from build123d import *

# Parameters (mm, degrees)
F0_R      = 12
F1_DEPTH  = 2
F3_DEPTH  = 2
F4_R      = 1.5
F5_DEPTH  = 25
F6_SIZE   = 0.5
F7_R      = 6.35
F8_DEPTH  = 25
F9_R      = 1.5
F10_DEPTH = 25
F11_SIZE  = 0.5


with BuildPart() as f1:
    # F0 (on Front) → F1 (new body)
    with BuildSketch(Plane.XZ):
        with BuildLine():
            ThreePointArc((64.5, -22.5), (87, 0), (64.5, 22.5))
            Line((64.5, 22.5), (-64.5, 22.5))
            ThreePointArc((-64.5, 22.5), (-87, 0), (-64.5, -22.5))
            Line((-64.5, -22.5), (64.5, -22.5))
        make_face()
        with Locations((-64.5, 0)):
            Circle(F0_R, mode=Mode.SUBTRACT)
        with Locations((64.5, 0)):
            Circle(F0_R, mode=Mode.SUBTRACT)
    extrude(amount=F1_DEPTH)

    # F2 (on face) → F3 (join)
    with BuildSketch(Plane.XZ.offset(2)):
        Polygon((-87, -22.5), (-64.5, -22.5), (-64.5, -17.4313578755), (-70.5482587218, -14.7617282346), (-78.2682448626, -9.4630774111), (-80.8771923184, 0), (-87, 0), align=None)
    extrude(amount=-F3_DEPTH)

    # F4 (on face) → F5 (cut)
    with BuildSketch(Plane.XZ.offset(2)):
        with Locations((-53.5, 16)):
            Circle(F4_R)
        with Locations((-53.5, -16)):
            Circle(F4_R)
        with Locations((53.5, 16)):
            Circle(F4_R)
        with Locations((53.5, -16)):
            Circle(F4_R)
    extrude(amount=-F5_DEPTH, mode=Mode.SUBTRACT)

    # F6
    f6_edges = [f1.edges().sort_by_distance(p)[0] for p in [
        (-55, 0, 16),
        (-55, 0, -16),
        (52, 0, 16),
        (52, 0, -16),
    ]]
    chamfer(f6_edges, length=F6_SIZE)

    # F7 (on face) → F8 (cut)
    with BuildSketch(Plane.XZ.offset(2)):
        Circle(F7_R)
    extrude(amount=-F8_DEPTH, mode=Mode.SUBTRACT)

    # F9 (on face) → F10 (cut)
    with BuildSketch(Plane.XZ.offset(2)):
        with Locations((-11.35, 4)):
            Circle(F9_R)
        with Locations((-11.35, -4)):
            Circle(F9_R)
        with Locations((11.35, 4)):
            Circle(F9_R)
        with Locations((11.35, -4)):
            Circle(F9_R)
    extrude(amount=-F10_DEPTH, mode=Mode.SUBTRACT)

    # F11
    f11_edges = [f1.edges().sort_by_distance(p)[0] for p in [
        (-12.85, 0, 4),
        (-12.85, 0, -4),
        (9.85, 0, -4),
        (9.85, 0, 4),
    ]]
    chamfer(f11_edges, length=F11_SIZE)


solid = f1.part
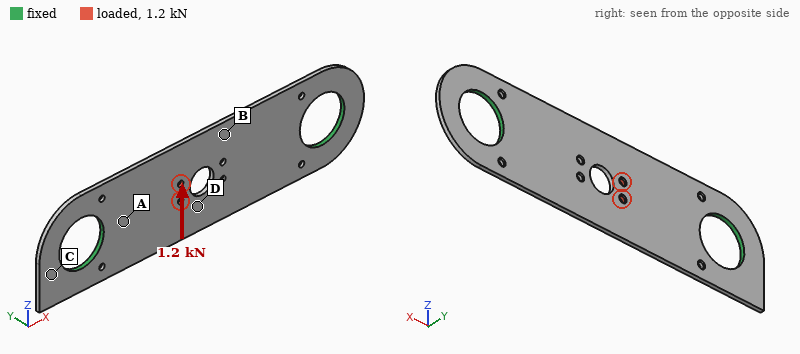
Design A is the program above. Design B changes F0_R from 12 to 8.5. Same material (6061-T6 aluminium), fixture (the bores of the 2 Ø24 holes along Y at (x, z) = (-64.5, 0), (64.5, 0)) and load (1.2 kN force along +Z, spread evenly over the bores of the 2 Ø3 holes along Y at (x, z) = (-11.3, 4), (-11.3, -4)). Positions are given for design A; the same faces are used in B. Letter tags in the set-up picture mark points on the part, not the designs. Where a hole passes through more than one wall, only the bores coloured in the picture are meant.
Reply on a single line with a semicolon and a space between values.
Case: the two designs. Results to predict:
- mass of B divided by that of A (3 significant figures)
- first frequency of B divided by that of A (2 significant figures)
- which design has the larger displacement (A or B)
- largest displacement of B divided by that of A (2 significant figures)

1.07; 0.87; B; 1.2
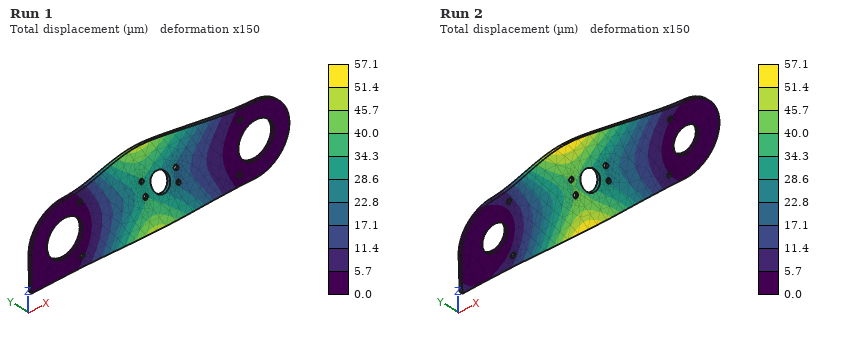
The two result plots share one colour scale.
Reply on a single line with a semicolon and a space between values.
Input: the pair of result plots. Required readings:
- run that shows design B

Run 2
